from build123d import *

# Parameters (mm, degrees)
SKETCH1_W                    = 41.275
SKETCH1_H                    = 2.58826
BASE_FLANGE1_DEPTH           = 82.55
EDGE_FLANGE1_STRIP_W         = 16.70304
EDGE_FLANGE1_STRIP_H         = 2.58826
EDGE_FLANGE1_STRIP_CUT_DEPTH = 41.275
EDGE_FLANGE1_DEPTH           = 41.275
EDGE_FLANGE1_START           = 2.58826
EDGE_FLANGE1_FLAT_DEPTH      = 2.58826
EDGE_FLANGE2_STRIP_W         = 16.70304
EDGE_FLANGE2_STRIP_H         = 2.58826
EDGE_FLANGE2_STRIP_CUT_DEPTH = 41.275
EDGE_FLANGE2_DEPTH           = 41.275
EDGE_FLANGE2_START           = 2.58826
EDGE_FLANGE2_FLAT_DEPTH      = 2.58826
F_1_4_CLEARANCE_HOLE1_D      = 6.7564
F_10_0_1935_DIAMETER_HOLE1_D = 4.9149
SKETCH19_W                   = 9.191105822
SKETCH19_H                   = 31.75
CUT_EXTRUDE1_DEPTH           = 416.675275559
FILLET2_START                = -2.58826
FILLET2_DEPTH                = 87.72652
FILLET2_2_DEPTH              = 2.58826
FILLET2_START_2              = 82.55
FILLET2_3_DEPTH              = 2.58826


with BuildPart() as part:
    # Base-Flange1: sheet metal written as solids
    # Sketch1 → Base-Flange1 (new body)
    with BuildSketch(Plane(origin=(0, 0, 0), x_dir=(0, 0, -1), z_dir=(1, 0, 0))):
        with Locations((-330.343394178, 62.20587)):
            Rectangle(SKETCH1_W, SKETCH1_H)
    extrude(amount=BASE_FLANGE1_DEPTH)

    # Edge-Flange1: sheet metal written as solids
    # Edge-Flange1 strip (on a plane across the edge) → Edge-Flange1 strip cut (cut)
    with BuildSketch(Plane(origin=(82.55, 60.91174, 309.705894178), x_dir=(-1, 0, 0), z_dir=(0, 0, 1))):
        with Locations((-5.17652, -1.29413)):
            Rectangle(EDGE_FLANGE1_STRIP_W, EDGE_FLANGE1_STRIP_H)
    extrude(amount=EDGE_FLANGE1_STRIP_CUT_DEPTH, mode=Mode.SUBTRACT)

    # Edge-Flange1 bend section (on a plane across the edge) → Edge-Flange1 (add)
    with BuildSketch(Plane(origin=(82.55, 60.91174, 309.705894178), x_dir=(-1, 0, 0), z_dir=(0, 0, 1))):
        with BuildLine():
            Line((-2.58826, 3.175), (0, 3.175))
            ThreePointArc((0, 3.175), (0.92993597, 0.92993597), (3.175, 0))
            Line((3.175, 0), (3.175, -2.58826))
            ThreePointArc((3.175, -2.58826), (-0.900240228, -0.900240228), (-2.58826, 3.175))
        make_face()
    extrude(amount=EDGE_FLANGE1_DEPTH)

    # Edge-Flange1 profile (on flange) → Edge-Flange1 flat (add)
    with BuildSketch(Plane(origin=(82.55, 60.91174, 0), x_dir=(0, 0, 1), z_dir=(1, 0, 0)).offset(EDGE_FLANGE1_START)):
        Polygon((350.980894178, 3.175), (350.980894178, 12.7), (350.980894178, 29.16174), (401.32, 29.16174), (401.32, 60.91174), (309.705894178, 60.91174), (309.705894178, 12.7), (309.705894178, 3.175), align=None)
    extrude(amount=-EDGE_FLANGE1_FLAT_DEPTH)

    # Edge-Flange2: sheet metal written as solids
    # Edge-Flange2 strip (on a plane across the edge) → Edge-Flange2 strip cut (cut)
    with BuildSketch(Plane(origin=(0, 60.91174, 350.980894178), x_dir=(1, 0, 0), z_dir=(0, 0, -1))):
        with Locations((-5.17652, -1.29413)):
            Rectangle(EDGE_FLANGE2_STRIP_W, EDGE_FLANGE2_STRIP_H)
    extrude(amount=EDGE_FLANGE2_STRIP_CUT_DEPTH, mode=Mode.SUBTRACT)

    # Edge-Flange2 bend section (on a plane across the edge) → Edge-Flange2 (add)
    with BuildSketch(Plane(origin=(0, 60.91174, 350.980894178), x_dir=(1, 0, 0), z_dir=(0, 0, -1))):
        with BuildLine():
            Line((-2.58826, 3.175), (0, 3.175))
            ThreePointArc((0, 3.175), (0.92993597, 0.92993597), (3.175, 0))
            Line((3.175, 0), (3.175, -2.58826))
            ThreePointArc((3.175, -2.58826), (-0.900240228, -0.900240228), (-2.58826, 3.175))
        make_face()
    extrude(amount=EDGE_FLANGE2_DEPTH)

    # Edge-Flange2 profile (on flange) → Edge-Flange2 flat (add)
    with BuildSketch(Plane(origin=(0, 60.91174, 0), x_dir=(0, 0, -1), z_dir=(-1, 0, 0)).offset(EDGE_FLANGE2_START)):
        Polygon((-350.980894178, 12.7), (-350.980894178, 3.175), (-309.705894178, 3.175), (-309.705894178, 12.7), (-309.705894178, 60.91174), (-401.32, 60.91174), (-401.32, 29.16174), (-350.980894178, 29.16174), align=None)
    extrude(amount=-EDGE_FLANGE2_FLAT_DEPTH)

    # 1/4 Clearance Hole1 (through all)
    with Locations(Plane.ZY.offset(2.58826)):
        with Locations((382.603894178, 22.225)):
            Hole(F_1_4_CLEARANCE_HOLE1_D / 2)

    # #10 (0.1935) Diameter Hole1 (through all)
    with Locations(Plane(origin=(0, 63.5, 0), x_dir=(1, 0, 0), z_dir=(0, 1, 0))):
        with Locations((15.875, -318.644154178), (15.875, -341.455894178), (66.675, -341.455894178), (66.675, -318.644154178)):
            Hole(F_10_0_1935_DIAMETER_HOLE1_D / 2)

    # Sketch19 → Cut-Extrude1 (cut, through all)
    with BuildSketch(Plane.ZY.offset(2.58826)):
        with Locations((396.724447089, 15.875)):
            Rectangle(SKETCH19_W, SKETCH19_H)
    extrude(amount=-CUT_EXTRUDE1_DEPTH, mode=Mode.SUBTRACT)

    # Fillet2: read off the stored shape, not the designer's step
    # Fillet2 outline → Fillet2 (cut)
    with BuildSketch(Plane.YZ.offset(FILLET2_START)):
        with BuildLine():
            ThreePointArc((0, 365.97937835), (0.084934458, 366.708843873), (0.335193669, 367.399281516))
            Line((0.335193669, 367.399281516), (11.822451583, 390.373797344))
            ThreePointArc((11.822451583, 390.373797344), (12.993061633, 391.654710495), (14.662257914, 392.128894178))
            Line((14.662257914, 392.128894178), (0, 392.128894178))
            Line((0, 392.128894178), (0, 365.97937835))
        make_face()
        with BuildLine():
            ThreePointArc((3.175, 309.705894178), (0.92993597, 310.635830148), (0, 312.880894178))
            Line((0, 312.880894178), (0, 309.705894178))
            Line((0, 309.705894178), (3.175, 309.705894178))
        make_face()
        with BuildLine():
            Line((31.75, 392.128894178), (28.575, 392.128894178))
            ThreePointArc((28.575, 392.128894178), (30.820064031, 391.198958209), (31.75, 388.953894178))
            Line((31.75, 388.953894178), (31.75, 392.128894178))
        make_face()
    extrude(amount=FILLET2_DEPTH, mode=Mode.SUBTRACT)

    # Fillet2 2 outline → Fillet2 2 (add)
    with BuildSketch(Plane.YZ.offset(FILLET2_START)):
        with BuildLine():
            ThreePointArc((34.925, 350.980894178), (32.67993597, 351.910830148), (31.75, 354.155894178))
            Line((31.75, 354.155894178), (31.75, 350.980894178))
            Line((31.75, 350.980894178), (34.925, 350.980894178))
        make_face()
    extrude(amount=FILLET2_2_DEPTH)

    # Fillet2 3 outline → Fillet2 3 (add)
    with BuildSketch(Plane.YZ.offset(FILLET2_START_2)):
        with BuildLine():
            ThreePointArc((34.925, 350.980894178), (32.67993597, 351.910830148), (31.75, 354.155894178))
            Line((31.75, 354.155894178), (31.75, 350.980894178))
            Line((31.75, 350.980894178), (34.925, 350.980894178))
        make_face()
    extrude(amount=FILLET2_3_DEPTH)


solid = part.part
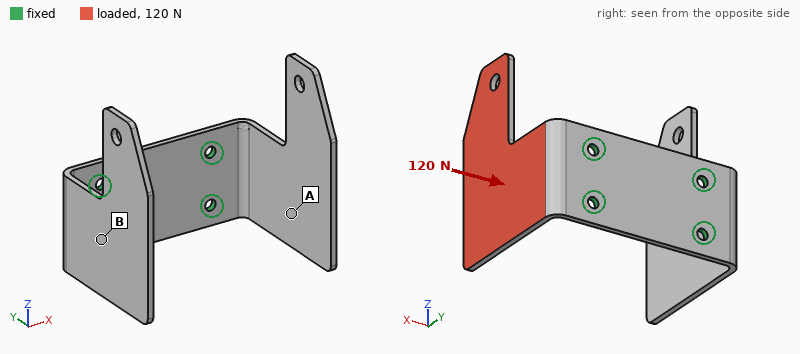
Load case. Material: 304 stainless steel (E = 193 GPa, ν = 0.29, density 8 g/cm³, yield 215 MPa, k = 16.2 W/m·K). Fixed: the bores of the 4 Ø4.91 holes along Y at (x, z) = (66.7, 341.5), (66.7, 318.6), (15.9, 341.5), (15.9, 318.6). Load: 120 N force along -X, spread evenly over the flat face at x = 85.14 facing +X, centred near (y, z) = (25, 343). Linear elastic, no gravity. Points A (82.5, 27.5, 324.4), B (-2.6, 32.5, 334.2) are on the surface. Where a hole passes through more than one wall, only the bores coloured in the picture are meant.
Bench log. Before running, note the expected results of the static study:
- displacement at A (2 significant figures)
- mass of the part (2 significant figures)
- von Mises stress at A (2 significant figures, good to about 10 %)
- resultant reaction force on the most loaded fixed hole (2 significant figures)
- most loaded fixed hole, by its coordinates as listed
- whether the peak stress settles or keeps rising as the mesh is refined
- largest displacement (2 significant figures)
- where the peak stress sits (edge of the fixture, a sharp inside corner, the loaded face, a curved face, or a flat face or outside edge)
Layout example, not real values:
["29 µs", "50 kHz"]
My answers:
["0.32 mm", "220 g", "26 MPa", "110 N", "(66.7, 341.5)", "keeps rising", "0.83 mm", "edge of the fixture"]
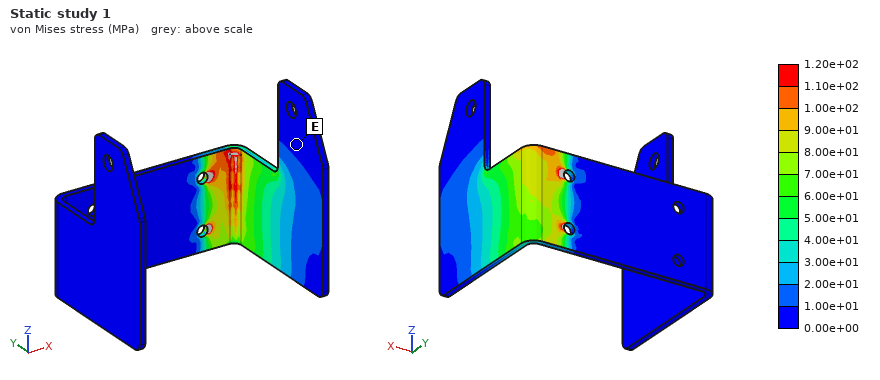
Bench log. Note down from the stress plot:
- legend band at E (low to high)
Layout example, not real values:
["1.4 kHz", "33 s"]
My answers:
["0.00e+00 to 1.00e+01 MPa"]
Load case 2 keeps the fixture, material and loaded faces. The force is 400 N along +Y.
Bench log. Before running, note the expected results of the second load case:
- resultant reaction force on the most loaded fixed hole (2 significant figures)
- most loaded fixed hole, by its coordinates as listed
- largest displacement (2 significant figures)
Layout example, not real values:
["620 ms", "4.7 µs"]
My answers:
["390 N", "(66.7, 341.5)", "0.46 mm"]
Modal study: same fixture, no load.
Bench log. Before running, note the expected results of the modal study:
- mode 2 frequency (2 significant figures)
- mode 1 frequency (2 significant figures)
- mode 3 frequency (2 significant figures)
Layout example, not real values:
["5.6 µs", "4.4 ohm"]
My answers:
["280 Hz", "280 Hz", "600 Hz"]
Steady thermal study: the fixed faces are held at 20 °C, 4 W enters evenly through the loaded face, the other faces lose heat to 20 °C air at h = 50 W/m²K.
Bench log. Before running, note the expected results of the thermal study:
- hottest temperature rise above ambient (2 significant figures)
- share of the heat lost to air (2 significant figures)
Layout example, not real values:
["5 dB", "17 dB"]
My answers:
["18 K", "87 %"]
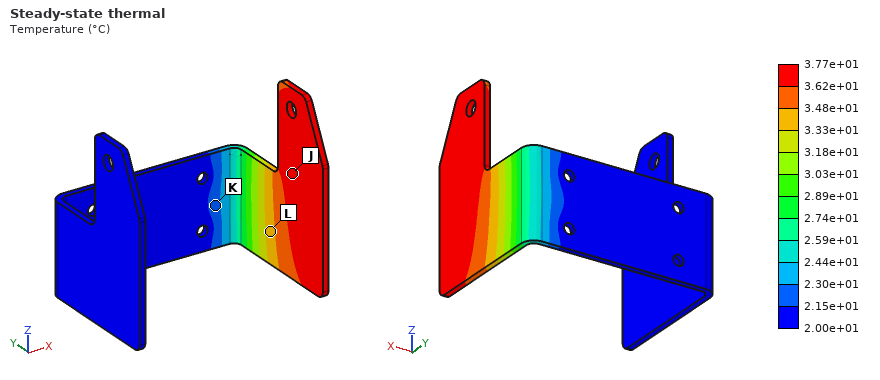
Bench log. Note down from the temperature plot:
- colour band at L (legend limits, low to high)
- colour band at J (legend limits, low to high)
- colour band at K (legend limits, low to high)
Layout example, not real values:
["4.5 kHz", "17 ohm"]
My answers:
["3.33e+01 to 3.48e+01 °C", "3.62e+01 to 3.77e+01 °C", "2.15e+01 to 2.30e+01 °C"]
